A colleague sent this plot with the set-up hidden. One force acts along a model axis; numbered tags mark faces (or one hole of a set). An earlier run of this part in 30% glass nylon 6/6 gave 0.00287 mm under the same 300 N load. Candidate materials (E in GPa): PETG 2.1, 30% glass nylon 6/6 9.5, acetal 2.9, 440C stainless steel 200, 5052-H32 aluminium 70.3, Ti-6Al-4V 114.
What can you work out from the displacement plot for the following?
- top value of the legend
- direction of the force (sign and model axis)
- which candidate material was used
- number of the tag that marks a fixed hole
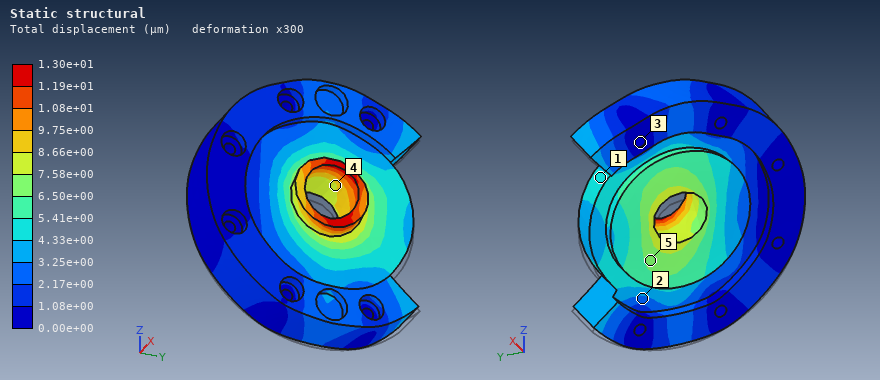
1.30e+01 µm
+Z
PETG
3
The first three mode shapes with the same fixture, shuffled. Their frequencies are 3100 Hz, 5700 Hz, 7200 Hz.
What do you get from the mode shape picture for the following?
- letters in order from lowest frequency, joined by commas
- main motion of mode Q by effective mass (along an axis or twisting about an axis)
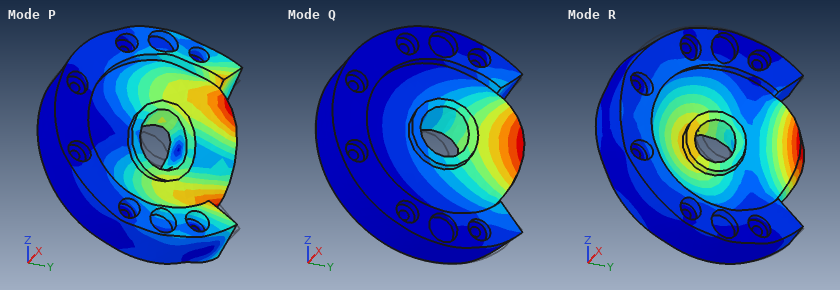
Q, R, P
along X
